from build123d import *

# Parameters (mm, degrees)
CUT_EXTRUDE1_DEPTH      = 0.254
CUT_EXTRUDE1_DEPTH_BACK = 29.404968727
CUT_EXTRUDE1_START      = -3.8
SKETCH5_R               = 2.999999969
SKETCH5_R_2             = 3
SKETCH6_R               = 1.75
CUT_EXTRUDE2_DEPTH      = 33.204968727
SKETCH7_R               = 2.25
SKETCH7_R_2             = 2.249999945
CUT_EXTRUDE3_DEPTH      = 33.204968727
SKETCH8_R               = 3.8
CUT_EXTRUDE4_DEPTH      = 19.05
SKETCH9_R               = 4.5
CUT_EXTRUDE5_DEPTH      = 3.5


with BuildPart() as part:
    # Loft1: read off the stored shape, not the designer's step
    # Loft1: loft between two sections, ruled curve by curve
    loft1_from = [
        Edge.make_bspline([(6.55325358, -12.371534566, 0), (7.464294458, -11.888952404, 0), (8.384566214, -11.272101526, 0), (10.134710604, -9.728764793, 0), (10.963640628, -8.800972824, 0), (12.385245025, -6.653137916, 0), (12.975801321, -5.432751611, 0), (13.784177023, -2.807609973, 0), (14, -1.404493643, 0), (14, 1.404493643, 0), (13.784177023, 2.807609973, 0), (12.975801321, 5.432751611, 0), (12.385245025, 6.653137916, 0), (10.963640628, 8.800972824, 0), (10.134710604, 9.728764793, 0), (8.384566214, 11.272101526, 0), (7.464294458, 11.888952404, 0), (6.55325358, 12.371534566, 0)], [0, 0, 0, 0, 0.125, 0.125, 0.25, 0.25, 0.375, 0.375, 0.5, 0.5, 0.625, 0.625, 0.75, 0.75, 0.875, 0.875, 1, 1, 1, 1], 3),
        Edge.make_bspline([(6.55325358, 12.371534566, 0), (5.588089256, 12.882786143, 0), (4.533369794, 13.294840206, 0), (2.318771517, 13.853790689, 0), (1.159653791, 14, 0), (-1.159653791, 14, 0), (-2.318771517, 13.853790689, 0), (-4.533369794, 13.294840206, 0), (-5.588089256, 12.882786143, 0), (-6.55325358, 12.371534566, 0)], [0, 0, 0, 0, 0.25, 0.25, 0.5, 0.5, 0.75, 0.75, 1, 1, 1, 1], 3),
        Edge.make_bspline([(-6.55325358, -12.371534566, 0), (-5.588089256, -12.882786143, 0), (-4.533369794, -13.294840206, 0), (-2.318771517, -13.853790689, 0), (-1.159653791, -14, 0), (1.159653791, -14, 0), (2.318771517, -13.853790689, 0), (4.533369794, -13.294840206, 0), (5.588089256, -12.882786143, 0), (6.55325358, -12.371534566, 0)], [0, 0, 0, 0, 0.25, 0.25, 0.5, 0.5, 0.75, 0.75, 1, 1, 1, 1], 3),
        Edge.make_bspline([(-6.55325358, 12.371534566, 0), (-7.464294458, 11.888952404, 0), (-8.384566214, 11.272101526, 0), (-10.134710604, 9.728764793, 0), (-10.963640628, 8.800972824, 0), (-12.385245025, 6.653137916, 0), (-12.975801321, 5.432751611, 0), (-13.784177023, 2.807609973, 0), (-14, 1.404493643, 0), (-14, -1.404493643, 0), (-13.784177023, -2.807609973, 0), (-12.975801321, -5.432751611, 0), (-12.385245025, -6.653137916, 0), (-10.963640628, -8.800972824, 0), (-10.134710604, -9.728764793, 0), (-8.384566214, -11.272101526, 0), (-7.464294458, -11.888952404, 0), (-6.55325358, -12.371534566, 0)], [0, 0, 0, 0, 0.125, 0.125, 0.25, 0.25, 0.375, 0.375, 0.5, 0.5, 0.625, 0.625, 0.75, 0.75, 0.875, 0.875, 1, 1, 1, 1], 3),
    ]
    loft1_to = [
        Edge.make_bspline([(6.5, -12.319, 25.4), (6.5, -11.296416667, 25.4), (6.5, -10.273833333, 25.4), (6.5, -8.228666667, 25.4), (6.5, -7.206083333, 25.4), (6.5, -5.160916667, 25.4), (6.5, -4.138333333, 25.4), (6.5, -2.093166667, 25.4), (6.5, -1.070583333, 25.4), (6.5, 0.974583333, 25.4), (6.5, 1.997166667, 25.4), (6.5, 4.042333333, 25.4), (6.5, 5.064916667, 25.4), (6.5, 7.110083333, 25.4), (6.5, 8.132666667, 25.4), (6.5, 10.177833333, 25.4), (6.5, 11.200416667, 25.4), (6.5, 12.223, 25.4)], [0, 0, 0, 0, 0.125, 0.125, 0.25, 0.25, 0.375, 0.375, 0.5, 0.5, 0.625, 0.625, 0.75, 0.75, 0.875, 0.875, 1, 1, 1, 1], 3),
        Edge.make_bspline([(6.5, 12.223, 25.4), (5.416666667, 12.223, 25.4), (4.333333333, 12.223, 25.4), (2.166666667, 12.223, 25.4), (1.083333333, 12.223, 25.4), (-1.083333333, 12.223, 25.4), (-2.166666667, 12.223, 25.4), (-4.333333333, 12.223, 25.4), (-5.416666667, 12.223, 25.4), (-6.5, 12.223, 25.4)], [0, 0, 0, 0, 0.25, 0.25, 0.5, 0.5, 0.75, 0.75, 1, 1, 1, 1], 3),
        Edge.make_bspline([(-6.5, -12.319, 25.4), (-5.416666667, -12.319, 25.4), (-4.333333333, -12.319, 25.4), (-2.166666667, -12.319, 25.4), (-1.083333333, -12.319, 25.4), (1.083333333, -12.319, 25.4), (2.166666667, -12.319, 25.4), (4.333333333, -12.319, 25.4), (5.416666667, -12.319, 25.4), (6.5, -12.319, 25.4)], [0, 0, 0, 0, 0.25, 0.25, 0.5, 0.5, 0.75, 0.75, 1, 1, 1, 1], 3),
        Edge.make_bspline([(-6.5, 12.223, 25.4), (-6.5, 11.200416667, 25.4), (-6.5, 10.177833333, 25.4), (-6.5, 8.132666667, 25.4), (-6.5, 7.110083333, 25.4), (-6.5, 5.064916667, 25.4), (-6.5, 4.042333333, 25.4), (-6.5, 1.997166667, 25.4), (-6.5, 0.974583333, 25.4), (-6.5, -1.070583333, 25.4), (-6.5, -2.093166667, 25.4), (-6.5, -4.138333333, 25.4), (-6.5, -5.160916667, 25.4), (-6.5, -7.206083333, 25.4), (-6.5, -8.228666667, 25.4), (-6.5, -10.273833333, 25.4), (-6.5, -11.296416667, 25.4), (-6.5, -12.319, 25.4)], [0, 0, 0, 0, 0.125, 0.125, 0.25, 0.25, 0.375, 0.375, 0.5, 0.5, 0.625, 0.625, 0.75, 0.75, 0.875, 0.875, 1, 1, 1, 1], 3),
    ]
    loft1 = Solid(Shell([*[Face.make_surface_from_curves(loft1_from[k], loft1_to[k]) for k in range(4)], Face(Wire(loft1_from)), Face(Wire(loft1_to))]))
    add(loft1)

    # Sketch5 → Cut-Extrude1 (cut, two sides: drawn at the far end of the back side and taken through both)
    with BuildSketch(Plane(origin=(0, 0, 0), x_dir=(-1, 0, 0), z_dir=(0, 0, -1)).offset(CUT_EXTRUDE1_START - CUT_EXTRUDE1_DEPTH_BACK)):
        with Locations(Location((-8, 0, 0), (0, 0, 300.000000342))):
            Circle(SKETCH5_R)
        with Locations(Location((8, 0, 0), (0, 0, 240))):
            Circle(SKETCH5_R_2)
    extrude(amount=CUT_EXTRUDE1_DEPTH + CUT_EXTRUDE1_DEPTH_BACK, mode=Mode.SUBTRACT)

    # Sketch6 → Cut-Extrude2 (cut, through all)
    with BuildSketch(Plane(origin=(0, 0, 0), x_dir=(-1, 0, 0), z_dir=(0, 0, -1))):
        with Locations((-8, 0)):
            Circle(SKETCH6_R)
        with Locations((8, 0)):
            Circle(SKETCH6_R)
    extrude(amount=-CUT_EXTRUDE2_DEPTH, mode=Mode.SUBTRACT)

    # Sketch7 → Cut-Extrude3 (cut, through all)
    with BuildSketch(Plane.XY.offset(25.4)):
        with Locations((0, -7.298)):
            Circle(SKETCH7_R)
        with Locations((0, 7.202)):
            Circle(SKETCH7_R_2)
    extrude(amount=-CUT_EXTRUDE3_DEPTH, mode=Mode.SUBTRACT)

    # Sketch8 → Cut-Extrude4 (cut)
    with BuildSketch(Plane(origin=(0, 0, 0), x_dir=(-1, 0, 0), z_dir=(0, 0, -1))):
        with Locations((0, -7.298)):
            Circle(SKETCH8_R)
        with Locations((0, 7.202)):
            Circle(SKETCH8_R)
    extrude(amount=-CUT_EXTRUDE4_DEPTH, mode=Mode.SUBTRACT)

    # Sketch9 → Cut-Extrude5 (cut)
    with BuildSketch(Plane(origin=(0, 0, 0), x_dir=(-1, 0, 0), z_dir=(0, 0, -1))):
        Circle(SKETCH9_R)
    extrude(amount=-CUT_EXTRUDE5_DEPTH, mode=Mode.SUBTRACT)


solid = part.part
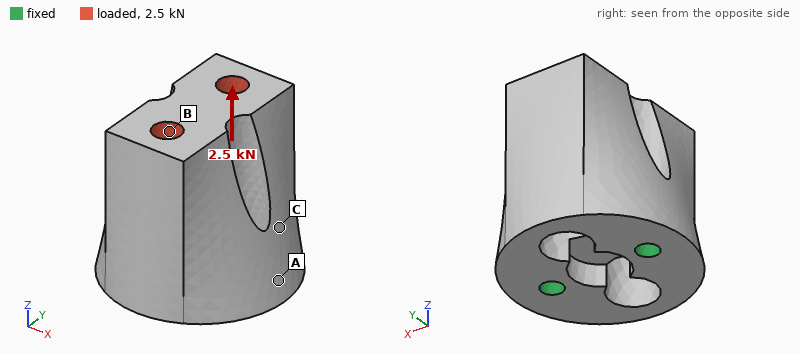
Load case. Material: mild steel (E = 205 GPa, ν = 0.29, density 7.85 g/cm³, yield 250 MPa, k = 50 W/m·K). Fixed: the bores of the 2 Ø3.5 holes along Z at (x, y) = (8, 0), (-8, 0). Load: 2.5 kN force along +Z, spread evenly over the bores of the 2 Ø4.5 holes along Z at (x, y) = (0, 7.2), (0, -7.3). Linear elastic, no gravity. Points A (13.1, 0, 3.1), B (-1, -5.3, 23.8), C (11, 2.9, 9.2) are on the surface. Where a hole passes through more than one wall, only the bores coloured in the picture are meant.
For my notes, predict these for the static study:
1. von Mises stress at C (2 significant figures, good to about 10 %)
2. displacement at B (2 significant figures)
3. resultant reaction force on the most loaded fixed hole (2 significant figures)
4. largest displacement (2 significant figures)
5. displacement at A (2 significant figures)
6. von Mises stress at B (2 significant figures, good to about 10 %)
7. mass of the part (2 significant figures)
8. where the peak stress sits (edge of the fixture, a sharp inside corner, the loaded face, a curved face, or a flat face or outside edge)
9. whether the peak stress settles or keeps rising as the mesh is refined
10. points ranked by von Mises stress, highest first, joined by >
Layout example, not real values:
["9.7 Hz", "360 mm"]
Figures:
["19 MPa", "2.6 µm", "1.3 kN", "2.9 µm", "0.63 µm", "31 MPa", "68 g", "edge of the fixture", "keeps rising", "B > C > A"]
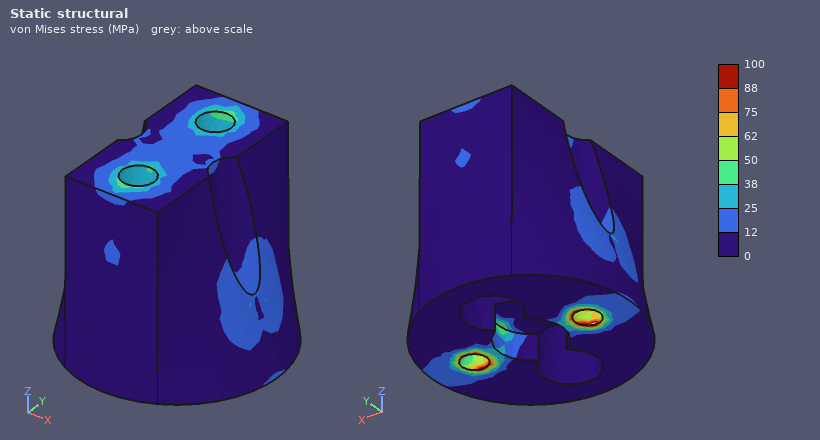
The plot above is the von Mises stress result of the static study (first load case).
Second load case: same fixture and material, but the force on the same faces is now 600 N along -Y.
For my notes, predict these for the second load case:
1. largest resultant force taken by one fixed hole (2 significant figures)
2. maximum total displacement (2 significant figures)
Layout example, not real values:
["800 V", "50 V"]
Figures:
["300 N", "21 µm"]
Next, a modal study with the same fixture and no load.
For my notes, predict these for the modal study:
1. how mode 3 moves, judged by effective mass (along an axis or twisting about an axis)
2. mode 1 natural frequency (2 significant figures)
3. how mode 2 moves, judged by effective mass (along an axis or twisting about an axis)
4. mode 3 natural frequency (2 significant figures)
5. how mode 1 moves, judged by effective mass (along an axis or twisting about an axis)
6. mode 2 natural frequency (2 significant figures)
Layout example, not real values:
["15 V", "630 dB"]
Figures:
["twisting about Z", "5400 Hz", "along X", "23 kHz", "along Y", "14 kHz"]
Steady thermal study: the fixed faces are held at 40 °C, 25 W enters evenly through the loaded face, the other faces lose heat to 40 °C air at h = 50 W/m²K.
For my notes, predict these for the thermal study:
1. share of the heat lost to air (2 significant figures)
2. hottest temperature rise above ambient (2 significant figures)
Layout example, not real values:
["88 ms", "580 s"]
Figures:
["19 %", "46 K"]
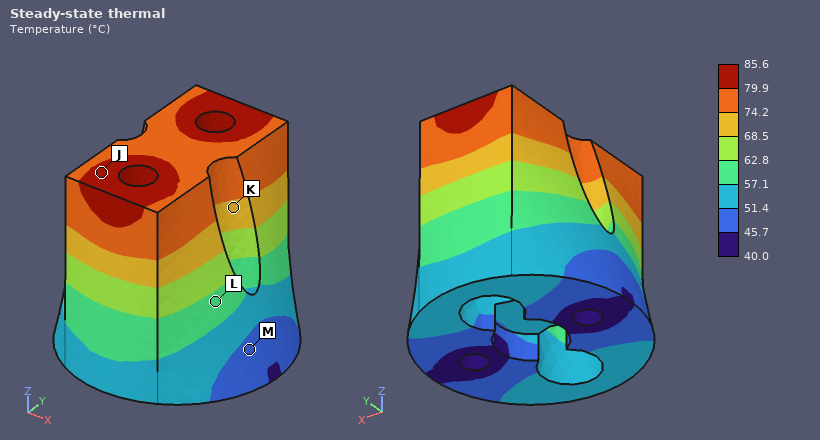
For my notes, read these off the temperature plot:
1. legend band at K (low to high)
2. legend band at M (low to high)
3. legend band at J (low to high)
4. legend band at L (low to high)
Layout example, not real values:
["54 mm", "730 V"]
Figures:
["68.5 to 74.2 °C", "45.7 to 51.4 °C", "79.9 to 85.6 °C", "57.1 to 62.8 °C"]
